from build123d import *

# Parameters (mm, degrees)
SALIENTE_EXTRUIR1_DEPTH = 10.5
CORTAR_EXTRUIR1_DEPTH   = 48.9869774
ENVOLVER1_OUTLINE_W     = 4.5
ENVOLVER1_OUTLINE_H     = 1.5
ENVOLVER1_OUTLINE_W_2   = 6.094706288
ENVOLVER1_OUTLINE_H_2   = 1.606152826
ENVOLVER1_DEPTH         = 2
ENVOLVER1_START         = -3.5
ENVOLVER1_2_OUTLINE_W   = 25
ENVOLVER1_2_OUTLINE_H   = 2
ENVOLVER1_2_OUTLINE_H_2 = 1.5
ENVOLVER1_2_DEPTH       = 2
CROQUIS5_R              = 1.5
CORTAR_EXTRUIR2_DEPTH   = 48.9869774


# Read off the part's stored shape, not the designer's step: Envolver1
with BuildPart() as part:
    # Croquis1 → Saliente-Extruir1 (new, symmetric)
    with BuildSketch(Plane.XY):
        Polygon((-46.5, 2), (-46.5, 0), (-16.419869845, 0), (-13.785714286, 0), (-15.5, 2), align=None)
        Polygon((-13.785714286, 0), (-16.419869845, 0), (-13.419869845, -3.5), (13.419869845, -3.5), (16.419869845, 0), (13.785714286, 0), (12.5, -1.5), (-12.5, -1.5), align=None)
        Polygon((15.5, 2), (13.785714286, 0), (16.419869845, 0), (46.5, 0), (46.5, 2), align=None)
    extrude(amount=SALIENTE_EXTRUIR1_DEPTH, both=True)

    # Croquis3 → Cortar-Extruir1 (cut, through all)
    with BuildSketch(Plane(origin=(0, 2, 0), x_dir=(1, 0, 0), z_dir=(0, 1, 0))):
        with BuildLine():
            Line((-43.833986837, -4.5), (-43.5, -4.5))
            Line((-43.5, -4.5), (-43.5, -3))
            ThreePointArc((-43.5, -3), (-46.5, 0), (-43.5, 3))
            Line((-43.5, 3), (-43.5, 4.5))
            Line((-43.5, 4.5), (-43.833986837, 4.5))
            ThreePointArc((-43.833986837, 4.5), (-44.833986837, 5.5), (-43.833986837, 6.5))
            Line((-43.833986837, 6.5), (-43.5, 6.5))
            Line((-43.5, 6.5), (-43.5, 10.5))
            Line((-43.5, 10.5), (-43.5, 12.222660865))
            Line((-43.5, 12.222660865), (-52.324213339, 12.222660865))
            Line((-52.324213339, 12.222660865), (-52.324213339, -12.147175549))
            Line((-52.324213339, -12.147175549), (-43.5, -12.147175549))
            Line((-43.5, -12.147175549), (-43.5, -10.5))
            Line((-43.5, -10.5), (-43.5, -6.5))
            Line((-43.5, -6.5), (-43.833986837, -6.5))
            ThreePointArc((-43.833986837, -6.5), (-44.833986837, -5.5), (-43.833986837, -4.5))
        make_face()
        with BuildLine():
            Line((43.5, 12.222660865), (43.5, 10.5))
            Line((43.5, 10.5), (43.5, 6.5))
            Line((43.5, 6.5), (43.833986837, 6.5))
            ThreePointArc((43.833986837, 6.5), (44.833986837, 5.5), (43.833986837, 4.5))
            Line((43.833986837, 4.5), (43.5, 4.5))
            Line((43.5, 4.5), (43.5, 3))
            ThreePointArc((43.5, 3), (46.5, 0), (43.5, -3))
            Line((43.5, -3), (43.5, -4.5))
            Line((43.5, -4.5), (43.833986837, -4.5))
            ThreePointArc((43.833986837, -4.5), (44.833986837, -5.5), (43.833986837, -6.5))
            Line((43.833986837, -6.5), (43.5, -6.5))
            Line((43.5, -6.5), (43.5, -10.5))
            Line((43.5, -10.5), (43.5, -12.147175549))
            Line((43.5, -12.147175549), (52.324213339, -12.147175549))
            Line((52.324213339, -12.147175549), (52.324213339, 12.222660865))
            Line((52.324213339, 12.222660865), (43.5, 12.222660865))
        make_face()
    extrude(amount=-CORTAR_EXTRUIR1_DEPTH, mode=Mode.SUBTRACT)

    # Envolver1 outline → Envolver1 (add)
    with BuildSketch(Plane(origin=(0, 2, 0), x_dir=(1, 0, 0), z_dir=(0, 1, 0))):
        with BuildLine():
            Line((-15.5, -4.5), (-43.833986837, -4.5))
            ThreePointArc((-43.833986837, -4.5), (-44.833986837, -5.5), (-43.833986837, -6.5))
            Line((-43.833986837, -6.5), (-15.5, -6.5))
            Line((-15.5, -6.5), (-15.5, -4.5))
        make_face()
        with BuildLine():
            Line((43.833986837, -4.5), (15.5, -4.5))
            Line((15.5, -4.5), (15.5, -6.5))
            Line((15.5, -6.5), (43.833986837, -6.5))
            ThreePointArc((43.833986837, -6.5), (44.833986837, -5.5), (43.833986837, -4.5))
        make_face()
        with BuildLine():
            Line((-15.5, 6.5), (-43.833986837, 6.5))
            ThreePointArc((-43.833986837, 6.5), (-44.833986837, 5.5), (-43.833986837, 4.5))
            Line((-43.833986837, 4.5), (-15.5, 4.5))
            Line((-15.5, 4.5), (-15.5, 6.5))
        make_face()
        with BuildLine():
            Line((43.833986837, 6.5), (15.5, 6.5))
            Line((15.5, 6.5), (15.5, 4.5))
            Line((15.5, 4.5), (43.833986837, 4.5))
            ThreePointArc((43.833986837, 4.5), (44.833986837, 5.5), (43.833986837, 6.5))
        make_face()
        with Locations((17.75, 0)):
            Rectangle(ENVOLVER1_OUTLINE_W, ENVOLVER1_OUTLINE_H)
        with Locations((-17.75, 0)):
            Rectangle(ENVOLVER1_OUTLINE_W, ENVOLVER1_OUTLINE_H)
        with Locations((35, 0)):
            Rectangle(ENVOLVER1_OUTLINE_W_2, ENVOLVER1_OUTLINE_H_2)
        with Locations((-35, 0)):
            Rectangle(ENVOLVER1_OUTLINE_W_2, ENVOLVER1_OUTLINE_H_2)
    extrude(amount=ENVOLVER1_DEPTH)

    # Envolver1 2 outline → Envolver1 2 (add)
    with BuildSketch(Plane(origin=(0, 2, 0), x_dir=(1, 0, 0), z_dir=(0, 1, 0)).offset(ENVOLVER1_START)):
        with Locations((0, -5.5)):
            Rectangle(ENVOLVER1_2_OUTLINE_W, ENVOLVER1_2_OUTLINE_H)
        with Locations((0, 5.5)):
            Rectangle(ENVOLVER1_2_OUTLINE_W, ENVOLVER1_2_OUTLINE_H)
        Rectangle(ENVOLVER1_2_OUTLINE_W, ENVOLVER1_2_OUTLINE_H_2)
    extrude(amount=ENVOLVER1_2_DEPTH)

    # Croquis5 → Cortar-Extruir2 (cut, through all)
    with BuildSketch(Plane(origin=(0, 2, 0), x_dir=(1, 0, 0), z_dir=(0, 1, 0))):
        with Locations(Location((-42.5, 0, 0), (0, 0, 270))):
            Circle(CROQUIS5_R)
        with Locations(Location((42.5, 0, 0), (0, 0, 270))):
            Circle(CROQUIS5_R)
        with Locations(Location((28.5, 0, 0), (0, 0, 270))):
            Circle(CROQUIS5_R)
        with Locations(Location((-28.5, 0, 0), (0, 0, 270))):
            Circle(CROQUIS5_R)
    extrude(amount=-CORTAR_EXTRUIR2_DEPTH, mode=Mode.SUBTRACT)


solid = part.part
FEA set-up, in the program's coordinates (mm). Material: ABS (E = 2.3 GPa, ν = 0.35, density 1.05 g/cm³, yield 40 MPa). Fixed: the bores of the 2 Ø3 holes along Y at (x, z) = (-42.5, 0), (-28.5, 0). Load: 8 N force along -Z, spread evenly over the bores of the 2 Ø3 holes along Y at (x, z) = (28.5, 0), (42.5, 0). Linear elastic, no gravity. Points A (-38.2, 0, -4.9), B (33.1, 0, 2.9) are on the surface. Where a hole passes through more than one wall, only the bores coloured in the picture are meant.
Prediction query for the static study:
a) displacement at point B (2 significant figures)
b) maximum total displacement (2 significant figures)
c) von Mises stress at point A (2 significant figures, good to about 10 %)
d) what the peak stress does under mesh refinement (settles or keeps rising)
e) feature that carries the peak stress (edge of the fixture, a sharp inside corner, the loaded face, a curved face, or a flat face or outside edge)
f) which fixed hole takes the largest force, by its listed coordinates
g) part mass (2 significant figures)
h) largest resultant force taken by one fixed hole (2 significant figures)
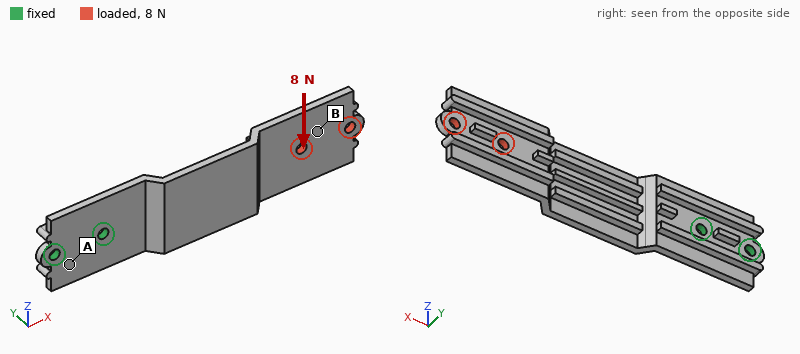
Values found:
0.67 mm
0.94 mm
1.8 MPa
keeps rising
a sharp inside corner
(-28.5, 0)
4.8 g
38 N
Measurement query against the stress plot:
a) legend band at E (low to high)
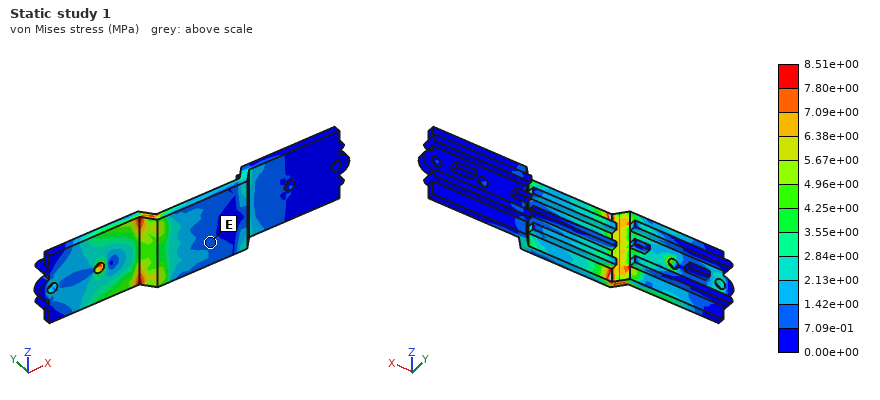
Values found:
7.09e-01 to 1.42e+00 MPa
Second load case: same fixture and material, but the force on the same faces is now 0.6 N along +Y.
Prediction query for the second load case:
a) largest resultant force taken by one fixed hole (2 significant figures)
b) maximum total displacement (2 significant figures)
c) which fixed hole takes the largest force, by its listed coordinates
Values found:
2.8 N
1.0 mm
(-28.5, 0)
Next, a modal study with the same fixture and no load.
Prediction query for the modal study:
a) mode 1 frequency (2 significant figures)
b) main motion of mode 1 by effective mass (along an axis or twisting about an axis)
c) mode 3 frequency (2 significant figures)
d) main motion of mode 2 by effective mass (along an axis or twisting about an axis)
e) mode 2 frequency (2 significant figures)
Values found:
120 Hz
along Y
700 Hz
along Z
410 Hz
